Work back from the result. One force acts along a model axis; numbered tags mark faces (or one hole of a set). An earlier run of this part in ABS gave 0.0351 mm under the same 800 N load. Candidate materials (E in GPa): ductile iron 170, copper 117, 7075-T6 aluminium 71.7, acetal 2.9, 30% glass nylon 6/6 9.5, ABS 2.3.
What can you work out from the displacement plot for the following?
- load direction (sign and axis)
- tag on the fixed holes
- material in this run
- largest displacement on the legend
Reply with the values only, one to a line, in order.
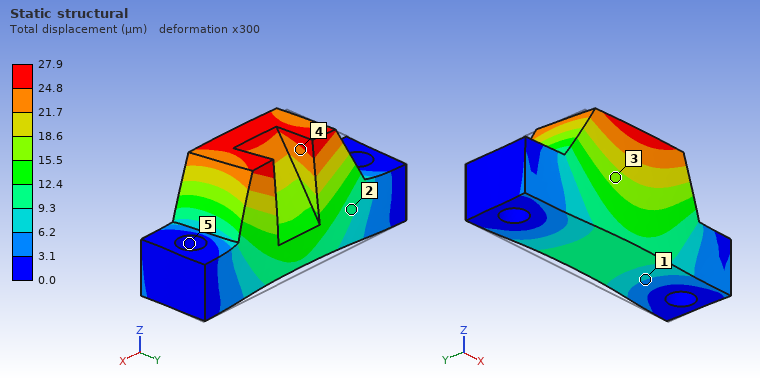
-Y
5
acetal
27.9 µm
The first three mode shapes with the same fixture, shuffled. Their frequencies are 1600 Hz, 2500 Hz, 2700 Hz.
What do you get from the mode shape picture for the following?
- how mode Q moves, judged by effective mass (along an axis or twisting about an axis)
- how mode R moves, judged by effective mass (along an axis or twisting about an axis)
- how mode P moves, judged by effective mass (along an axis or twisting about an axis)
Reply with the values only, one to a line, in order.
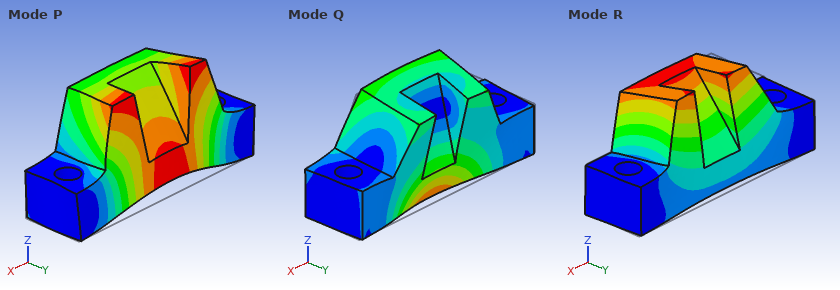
along Y
along Y
along Z
